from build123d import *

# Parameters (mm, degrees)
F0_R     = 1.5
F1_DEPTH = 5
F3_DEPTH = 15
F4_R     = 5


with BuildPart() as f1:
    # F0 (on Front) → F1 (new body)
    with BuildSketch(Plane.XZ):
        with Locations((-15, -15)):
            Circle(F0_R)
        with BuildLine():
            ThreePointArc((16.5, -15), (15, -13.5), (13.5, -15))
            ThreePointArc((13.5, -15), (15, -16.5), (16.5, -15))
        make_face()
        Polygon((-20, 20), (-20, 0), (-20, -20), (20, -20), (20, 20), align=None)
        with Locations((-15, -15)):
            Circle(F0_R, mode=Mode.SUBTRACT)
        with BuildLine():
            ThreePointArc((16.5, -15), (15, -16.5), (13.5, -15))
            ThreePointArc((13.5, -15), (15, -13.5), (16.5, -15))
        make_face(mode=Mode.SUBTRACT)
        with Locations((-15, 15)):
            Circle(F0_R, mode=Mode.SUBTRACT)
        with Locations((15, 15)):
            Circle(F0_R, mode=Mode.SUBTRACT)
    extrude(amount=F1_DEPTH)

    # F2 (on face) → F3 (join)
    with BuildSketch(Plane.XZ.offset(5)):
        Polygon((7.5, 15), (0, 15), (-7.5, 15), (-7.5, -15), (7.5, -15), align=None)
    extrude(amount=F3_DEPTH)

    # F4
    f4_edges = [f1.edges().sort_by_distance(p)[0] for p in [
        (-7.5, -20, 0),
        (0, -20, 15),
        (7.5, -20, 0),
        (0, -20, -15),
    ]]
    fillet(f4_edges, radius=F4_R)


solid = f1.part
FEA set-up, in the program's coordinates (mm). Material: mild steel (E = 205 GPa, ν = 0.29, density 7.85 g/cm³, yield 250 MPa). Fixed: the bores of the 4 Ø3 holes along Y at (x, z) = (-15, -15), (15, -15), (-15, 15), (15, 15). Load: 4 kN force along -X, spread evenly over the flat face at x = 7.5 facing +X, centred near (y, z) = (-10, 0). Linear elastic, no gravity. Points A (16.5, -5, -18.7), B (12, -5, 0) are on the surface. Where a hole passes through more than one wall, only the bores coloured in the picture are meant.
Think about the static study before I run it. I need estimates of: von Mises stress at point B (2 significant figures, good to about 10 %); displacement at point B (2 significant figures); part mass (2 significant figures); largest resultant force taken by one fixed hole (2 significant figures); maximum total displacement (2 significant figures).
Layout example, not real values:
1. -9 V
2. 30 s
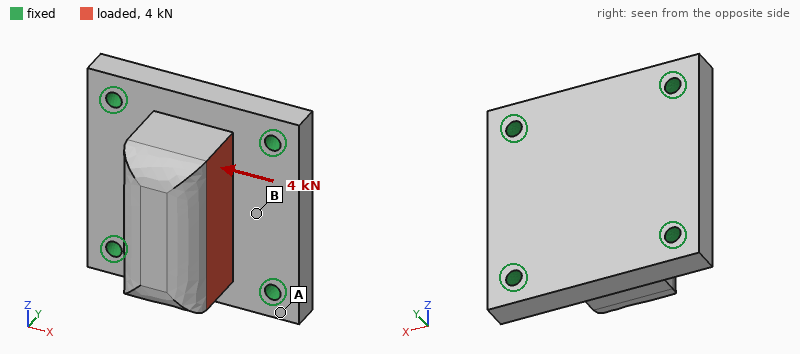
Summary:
1. 17 MPa
2. 2.6 µm
3. 110 g
4. 1.2 kN
5. 7.1 µm
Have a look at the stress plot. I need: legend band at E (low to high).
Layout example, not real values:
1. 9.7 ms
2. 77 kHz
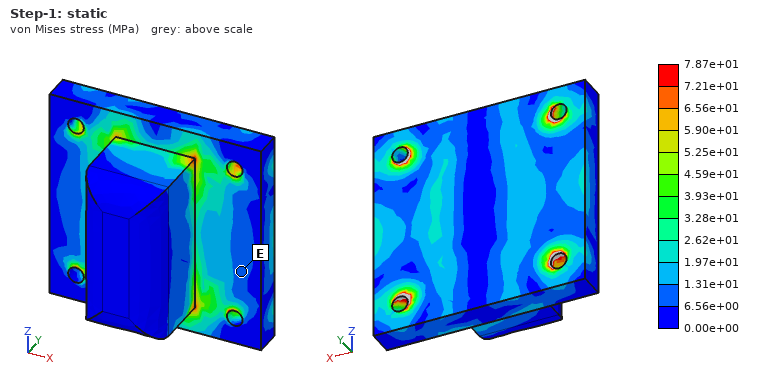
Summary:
1. 6.56e+00 to 1.31e+01 MPa
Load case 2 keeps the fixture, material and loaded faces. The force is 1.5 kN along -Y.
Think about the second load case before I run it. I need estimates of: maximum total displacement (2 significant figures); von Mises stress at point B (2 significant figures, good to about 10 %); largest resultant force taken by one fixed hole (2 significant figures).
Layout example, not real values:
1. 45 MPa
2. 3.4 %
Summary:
1. 4.0 µm
2. 12 MPa
3. 610 N
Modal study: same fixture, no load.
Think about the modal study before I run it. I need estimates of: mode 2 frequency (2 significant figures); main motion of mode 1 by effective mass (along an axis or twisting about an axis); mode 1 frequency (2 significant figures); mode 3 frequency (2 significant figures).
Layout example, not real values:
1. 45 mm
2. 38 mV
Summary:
1. 16 kHz
2. along Y
3. 14 kHz
4. 16 kHz
